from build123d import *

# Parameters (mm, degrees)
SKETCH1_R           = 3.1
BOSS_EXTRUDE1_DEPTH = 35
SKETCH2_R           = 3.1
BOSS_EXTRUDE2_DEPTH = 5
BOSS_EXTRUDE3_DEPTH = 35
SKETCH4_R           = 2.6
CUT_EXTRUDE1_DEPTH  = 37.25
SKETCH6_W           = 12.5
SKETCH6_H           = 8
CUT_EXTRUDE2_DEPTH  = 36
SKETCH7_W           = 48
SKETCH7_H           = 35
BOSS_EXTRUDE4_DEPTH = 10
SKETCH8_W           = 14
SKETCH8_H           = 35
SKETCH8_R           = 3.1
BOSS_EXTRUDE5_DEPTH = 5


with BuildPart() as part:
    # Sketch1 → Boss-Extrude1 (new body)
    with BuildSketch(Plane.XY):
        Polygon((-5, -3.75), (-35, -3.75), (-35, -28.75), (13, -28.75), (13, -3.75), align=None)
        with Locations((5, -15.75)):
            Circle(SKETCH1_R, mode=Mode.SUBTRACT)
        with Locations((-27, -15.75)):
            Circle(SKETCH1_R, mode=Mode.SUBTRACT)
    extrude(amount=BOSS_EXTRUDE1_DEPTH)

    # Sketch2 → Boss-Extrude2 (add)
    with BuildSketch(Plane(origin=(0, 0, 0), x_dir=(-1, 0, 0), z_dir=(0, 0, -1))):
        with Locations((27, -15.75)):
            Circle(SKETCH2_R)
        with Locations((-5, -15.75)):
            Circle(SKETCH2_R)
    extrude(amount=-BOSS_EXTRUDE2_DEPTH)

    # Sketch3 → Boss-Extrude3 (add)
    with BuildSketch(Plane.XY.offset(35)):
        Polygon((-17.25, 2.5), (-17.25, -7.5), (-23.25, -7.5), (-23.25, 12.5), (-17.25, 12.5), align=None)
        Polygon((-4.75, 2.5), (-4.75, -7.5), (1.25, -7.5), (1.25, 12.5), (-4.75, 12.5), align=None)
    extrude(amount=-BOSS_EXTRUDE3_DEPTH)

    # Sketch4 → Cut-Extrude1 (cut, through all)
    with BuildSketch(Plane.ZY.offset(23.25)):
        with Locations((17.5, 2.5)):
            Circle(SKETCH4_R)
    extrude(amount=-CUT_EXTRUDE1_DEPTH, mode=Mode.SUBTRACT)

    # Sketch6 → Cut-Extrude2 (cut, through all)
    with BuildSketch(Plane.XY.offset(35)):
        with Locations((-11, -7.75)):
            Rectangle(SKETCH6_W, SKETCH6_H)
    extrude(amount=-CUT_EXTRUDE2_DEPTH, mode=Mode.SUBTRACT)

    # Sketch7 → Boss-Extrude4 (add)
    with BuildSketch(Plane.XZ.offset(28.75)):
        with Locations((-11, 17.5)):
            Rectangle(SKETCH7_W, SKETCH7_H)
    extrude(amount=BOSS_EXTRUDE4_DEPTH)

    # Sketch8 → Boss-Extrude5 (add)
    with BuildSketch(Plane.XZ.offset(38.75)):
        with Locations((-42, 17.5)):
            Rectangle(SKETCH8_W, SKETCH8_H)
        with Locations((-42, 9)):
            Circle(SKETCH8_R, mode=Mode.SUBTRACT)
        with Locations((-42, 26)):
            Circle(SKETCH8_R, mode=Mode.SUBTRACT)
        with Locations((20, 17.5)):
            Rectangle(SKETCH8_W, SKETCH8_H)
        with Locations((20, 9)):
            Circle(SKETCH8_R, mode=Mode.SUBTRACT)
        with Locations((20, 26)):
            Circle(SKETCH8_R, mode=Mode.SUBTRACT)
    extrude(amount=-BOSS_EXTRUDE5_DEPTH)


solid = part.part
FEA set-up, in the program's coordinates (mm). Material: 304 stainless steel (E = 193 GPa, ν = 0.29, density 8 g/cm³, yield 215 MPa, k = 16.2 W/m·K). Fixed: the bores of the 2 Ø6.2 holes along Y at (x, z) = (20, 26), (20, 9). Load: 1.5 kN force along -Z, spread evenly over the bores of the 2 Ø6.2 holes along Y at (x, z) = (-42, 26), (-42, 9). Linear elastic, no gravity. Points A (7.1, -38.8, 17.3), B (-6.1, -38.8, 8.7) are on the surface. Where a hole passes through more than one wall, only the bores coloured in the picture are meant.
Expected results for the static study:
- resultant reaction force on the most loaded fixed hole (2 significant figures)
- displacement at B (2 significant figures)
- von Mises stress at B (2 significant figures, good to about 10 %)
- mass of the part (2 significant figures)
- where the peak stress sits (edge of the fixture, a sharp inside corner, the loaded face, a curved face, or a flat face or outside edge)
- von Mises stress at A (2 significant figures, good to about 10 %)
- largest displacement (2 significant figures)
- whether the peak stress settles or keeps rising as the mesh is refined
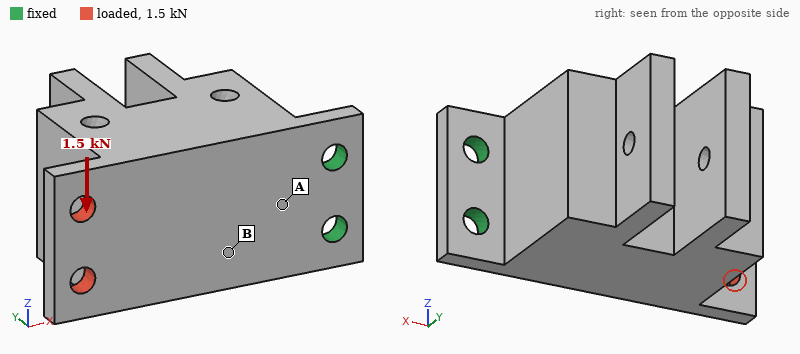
4.3 kN
13 µm
16 MPa
510 g
edge of the fixture
37 MPa
41 µm
keeps rising
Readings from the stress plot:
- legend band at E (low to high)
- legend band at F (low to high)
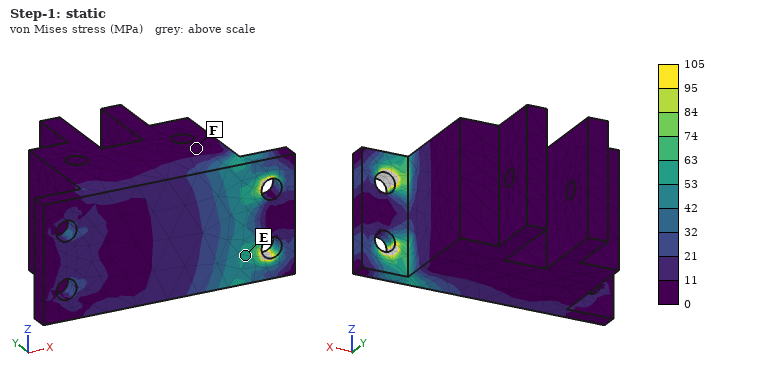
53 to 63 MPa
0 to 11 MPa
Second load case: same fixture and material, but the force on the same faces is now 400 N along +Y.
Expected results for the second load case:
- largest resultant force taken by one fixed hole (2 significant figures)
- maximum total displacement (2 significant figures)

200 N
0.17 mm
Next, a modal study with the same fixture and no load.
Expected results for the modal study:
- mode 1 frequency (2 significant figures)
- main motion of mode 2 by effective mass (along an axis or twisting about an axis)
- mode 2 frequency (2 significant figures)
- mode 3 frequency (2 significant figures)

580 Hz
along Z
2300 Hz
3600 Hz
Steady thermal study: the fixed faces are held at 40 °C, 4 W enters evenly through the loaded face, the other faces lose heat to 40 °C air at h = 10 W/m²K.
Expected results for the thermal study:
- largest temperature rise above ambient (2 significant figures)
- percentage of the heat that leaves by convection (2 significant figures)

36 K
46 %
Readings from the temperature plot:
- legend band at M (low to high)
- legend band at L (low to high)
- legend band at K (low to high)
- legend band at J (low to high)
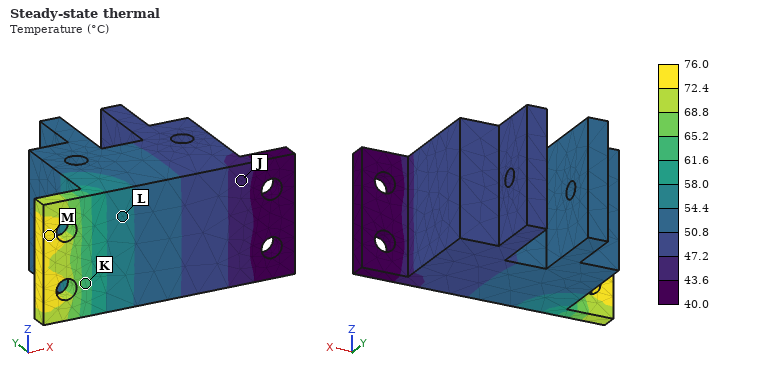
72.4 to 76.0 °C
54.4 to 58.0 °C
61.6 to 65.2 °C
43.6 to 47.2 °C
